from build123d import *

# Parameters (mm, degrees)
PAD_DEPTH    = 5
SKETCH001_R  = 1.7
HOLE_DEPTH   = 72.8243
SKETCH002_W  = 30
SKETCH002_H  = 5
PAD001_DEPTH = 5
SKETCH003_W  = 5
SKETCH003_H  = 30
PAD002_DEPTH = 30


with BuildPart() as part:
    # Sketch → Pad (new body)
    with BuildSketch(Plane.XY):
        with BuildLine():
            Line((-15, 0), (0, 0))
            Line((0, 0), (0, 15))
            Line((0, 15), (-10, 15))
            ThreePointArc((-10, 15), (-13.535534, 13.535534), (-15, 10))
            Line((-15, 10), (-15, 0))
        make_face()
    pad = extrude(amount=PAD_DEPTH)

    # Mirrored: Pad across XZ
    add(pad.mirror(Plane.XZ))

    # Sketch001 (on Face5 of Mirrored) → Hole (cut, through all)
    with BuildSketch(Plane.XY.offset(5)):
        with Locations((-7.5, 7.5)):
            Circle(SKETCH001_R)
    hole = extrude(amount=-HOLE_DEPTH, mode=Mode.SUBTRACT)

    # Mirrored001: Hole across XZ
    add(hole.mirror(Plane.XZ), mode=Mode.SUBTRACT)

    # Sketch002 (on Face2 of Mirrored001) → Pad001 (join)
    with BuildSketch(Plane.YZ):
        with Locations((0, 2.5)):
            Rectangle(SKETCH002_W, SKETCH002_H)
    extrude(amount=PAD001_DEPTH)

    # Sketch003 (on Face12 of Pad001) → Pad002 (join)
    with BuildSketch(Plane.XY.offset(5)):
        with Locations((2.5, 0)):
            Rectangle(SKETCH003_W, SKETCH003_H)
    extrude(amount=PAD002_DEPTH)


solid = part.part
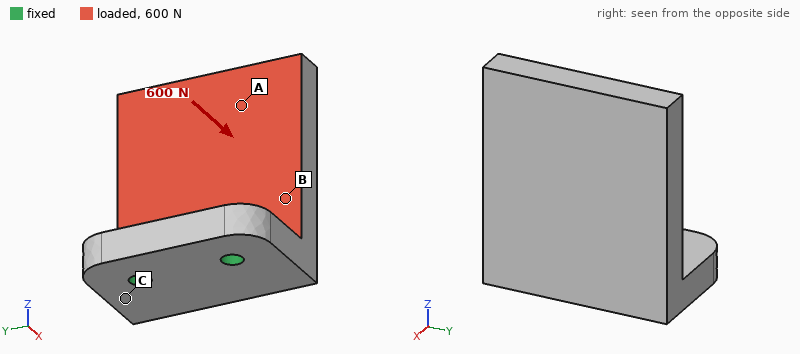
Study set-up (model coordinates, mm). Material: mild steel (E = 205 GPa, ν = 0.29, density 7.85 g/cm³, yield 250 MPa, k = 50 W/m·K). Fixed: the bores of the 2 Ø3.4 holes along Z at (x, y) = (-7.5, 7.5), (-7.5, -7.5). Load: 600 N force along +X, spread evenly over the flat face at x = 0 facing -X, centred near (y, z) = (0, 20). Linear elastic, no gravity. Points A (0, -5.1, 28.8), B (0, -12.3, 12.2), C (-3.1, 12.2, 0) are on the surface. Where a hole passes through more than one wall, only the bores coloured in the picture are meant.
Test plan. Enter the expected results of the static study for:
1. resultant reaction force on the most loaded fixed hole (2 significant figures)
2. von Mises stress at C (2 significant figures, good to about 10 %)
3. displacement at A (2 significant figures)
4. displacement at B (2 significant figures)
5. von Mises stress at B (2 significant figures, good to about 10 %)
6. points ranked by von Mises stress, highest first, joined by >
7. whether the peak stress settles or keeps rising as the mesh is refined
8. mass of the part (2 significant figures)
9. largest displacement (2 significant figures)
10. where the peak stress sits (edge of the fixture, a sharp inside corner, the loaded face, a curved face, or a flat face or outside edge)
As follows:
310 N
70 MPa
68 µm
19 µm
40 MPa
C > B > A
keeps rising
58 g
88 µm
edge of the fixture
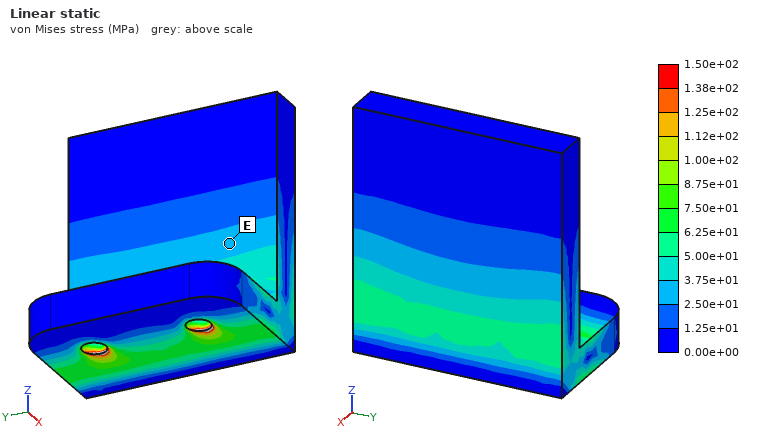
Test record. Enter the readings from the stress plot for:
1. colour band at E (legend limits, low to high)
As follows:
2.50e+01 to 3.75e+01 MPa
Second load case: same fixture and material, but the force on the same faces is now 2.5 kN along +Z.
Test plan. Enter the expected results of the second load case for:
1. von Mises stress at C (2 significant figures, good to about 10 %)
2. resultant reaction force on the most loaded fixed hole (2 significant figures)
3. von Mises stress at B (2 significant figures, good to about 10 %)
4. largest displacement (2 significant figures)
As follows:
44 MPa
1.3 kN
49 MPa
16 µm
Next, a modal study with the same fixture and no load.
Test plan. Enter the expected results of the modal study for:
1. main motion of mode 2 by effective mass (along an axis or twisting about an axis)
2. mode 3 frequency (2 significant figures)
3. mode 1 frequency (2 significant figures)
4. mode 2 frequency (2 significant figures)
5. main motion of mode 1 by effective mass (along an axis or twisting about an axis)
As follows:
along Y
9200 Hz
2700 Hz
5800 Hz
along X
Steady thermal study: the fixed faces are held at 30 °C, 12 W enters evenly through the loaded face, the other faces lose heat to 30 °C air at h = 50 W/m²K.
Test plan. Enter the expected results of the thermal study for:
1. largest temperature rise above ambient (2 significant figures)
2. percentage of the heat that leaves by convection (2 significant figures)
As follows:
34 K
19 %
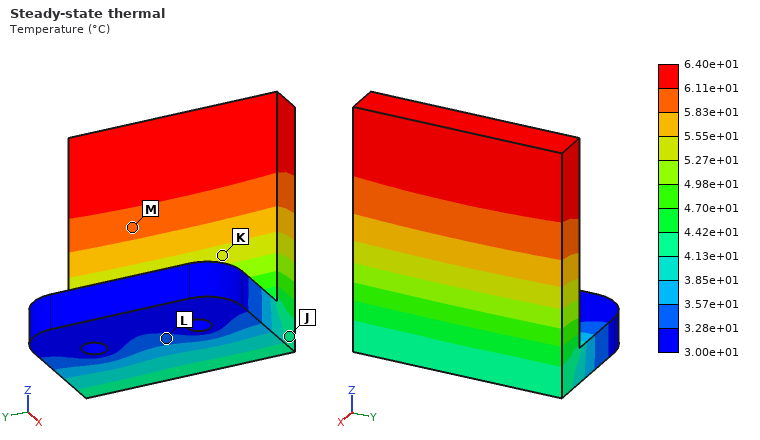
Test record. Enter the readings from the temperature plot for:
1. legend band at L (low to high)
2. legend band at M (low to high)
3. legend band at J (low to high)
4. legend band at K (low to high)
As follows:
3.28e+01 to 3.57e+01 °C
5.83e+01 to 6.11e+01 °C
4.13e+01 to 4.42e+01 °C
5.27e+01 to 5.55e+01 °C
